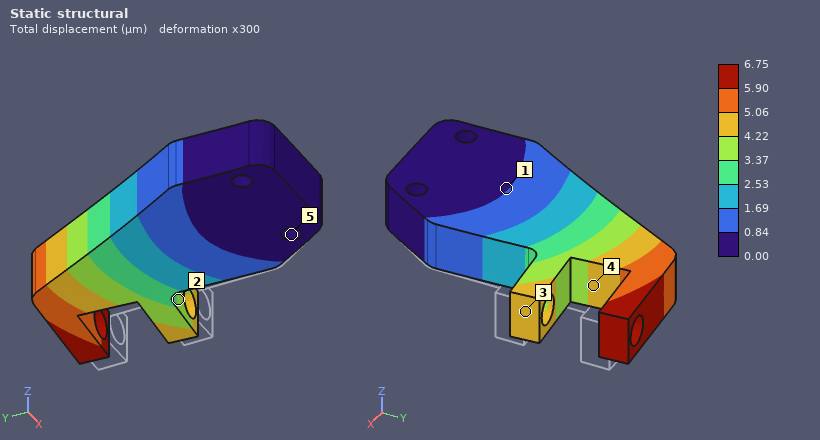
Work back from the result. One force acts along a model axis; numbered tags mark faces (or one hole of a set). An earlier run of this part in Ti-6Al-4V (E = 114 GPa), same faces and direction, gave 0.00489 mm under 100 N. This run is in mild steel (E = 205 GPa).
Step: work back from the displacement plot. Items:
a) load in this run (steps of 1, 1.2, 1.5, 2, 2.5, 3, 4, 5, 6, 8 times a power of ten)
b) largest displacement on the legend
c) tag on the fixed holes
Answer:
250 N
6.75 µm
5
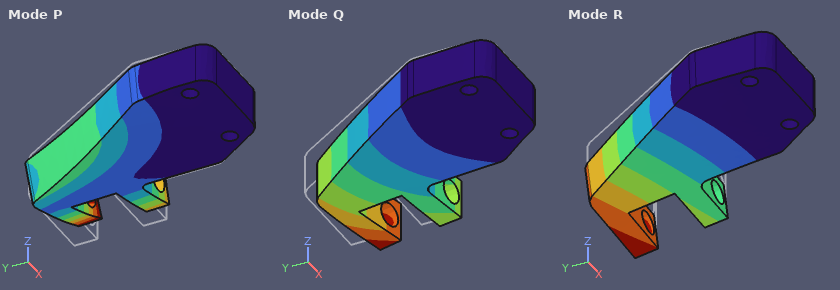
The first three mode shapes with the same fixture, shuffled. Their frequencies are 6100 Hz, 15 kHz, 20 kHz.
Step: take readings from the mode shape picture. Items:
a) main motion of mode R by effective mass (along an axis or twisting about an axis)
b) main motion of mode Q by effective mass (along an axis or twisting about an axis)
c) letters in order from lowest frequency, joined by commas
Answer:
along Z
along X
R, Q, P
